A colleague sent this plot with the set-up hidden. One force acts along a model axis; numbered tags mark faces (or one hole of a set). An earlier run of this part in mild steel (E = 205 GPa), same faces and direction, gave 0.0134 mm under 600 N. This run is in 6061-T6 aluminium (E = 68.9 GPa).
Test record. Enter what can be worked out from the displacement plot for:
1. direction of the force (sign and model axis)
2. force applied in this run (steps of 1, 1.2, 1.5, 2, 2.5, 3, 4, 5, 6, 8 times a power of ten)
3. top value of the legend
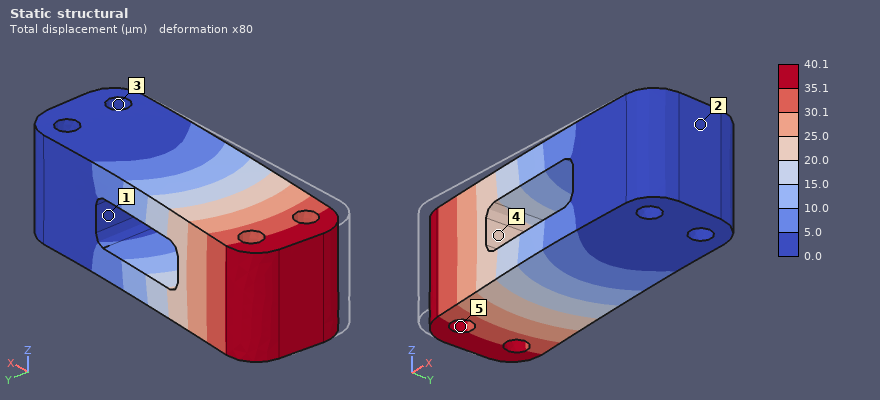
+Y
600 N
40.1 µm
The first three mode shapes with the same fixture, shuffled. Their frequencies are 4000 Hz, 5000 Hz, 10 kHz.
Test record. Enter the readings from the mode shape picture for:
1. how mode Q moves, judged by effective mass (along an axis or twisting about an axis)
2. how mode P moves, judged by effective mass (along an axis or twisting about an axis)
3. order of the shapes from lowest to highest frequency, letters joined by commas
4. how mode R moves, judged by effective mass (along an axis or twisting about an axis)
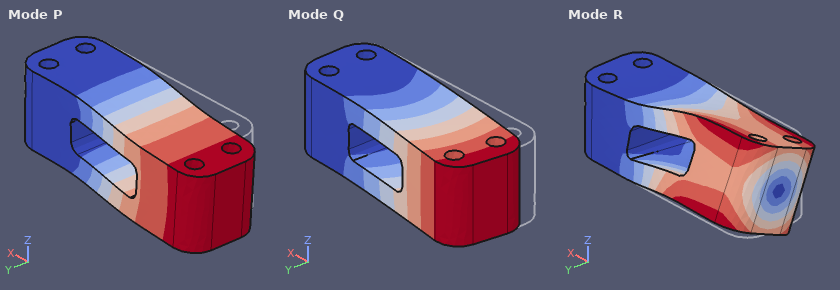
along Y
along Z
P, Q, R
twisting about X
